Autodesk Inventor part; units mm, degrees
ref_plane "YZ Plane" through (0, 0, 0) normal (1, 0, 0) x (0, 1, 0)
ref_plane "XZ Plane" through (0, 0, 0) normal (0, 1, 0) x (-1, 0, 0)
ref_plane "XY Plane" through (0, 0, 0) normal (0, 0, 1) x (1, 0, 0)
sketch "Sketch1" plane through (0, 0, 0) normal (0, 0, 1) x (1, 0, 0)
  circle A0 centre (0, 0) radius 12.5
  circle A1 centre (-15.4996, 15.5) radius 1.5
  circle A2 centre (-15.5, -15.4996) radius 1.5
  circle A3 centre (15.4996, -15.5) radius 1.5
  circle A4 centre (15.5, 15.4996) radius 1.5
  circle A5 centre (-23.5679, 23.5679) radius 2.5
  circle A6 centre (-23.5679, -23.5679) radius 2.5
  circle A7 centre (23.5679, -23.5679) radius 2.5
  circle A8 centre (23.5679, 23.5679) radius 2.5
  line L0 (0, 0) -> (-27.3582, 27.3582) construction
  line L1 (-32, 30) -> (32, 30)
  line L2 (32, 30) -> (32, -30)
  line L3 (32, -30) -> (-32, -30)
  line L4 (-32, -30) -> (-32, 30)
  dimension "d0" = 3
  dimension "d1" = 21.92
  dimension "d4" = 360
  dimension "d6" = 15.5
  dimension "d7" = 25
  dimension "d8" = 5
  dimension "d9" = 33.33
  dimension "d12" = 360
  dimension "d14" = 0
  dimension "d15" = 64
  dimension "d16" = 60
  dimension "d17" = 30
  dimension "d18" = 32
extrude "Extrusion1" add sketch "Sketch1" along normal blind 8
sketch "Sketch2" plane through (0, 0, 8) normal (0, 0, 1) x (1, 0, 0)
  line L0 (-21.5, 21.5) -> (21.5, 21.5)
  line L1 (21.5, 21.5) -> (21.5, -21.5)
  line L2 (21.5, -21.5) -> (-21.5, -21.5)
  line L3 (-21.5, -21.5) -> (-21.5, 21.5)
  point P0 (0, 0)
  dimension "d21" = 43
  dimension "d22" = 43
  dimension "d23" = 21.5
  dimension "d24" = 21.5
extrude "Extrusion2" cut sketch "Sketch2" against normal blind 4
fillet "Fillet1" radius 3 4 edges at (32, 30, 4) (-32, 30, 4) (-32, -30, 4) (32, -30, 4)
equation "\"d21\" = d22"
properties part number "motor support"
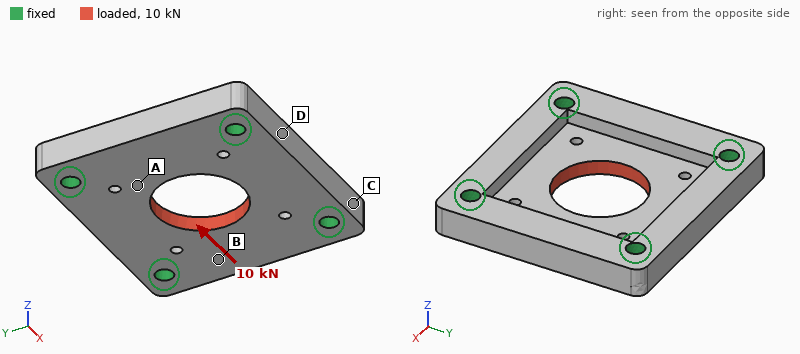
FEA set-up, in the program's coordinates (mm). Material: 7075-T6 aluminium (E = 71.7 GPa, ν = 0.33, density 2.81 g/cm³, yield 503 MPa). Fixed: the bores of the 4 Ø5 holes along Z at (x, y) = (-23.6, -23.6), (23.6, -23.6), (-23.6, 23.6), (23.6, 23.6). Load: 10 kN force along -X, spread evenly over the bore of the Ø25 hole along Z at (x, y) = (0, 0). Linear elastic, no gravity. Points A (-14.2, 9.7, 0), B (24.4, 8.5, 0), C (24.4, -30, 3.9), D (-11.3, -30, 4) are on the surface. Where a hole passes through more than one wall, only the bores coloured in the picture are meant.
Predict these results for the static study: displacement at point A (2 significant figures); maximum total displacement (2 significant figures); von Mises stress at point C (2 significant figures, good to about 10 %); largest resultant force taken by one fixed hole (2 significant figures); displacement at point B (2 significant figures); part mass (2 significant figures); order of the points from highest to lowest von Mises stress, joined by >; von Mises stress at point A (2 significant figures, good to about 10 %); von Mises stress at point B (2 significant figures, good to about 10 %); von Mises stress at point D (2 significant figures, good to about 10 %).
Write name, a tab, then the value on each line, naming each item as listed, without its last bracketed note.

displacement at point A	13 µm
maximum total displacement	19 µm
von Mises stress at point C	18 MPa
largest resultant force taken by one fixed hole	2.6 kN
displacement at point B	12 µm
part mass	58 g
order of the points from highest to lowest von Mises stress, joined by >	A > B > C > D
von Mises stress at point A	37 MPa
von Mises stress at point B	24 MPa
von Mises stress at point D	7.2 MPa
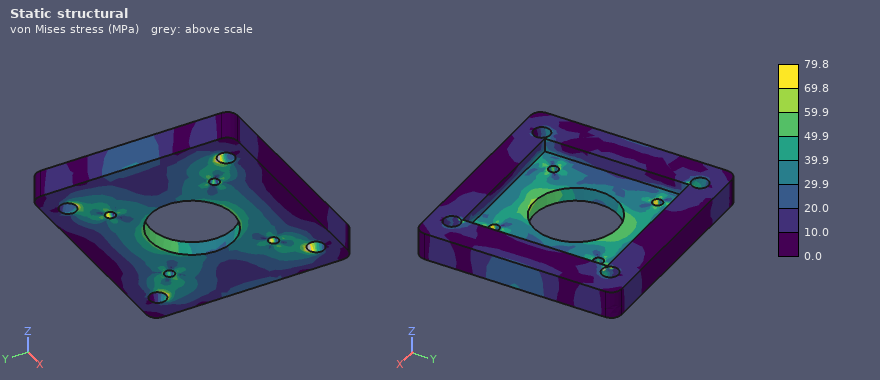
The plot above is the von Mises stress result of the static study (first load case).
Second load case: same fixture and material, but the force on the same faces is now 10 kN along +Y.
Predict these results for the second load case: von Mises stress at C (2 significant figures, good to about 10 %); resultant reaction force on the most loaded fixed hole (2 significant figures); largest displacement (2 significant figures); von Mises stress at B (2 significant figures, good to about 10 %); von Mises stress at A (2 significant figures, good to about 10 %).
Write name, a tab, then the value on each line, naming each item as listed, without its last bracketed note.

von Mises stress at C	24 MPa
resultant reaction force on the most loaded fixed hole	2.7 kN
largest displacement	20 µm
von Mises stress at B	14 MPa
von Mises stress at A	35 MPa
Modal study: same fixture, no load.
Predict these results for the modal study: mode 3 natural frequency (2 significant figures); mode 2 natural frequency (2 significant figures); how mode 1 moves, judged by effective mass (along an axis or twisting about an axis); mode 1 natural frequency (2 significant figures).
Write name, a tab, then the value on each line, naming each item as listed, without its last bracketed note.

mode 3 natural frequency	15 kHz
mode 2 natural frequency	15 kHz
how mode 1 moves, judged by effective mass	along Z
mode 1 natural frequency	13 kHz
